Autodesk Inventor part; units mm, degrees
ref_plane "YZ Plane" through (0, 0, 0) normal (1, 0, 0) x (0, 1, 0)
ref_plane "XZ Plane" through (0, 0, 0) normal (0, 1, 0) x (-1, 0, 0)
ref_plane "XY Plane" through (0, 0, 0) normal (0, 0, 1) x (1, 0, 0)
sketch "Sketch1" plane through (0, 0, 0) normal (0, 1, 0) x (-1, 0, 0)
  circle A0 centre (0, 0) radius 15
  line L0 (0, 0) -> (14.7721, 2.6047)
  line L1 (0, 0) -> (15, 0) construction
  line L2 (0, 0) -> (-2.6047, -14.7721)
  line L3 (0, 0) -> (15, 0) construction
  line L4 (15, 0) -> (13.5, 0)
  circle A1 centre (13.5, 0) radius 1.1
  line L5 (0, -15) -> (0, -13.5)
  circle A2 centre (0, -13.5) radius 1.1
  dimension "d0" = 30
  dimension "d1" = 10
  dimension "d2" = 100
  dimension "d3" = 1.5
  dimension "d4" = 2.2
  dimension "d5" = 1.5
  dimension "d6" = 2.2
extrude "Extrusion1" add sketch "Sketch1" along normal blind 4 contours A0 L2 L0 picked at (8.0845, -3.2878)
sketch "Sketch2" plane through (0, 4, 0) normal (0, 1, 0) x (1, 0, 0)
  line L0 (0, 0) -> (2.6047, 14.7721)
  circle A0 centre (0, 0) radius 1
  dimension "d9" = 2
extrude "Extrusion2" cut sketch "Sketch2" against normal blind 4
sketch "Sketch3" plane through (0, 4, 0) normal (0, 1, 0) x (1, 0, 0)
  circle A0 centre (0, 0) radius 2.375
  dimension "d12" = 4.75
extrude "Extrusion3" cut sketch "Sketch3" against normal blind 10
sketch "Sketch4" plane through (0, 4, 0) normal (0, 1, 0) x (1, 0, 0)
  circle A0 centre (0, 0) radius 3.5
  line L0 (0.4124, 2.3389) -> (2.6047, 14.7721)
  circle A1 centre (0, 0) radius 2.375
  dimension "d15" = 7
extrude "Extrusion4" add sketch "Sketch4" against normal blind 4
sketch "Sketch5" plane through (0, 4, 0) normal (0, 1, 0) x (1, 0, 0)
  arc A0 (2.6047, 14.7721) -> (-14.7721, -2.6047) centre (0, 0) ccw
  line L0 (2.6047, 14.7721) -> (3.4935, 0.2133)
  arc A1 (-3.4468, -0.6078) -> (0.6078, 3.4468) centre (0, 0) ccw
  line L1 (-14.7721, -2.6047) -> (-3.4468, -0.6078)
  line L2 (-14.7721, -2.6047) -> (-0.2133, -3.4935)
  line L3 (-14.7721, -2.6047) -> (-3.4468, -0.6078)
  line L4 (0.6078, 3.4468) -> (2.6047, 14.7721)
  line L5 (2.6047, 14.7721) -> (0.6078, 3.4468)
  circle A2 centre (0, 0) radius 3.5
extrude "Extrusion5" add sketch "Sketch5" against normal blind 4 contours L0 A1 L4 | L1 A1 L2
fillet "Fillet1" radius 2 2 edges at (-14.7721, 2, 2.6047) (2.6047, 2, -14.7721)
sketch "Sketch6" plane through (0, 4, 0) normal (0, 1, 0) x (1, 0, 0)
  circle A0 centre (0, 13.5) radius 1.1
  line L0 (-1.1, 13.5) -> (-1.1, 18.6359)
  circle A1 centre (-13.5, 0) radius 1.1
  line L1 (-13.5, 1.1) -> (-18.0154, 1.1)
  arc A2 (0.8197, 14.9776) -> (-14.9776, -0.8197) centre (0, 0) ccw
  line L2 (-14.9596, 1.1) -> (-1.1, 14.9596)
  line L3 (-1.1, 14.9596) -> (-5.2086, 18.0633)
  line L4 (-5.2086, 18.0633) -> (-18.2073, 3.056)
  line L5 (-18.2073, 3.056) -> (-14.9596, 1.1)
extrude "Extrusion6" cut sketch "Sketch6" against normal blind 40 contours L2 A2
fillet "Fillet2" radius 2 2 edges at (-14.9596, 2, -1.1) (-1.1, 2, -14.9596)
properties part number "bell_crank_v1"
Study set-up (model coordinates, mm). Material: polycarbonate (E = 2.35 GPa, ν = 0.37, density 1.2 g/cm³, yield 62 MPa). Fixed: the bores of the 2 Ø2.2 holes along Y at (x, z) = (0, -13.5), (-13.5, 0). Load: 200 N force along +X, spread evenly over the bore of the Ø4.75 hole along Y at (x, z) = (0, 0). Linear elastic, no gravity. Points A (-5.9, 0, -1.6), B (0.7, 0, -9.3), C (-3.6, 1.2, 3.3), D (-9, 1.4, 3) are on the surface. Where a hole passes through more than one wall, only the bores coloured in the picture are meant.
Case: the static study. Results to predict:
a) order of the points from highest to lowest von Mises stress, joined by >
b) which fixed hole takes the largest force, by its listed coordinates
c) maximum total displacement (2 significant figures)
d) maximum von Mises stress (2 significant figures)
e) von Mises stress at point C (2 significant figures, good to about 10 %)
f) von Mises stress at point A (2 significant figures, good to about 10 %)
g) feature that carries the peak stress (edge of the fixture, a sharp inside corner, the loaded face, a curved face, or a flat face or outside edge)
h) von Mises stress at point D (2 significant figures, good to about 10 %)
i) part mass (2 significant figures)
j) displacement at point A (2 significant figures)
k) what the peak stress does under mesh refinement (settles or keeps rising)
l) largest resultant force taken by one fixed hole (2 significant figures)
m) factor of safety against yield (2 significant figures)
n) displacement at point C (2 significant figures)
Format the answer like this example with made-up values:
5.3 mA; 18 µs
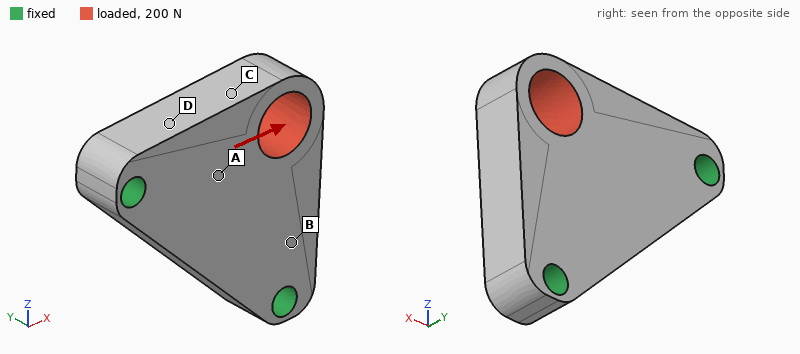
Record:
C > D > A > B; (-13.5, 0); 96 µm; 29 MPa; 17 MPa; 5.0 MPa; the loaded face; 9.6 MPa; 0.97 g; 24 µm; settles; 180 N; 2.1; 44 µm
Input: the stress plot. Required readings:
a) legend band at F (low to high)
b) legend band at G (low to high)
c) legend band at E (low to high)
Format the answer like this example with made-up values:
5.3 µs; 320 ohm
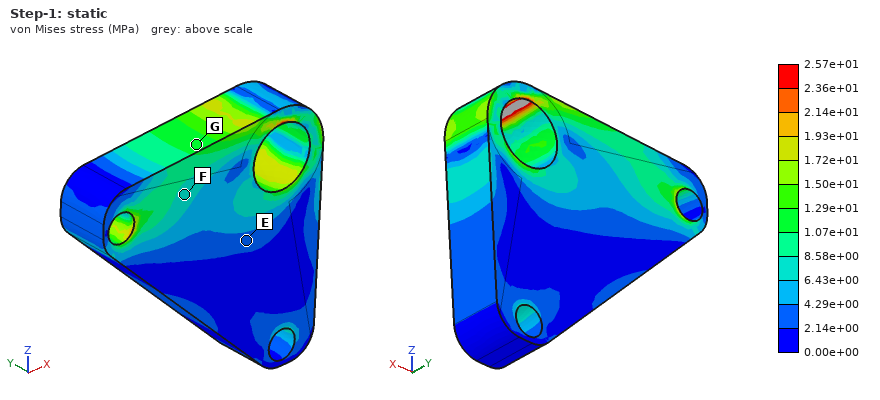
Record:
6.43e+00 to 8.58e+00 MPa; 1.07e+01 to 1.29e+01 MPa; 2.14e+00 to 4.29e+00 MPa
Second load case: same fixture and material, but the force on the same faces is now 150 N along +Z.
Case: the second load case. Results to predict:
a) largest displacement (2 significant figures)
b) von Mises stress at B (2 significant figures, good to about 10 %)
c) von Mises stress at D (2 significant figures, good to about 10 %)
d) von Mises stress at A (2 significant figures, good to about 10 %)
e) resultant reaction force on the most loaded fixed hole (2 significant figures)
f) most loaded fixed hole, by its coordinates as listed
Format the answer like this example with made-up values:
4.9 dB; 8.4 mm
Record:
72 µm; 6.7 MPa; 1.7 MPa; 1.6 MPa; 140 N; (0, -13.5)
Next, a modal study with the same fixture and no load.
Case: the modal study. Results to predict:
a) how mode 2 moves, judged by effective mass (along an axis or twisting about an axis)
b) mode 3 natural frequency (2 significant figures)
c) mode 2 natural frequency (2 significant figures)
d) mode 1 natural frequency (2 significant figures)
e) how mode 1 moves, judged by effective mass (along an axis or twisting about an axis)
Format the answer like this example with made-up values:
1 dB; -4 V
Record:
along Y; 15 kHz; 14 kHz; 5800 Hz; along Y
